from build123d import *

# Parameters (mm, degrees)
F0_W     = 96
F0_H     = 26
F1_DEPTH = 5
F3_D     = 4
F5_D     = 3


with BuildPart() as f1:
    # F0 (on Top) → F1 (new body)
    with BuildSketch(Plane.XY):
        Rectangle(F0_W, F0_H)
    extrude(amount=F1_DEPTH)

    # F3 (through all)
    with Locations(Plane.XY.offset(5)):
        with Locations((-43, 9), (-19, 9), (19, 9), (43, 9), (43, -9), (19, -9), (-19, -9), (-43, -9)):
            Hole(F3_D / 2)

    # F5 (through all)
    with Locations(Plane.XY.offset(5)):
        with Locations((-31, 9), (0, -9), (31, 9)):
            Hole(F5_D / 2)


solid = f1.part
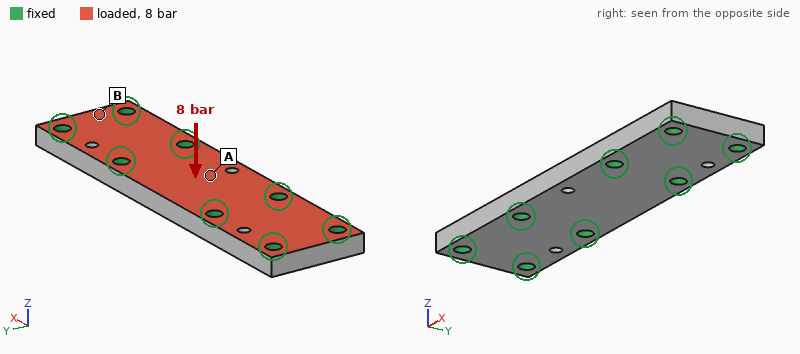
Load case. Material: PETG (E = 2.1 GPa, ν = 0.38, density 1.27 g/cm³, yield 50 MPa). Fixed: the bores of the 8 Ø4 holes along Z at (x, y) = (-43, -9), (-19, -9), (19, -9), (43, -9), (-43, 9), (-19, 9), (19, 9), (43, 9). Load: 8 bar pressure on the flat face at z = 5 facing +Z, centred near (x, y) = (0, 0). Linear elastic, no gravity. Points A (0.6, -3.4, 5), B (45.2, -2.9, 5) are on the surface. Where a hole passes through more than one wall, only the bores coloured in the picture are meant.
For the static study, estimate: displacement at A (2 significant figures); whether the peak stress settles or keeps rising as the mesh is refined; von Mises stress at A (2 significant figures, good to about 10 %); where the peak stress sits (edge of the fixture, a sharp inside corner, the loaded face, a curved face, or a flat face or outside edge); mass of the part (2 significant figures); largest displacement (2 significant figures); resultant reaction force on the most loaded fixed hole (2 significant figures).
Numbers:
0.21 mm
keeps rising
9.7 MPa
edge of the fixture
15 g
0.23 mm
320 N
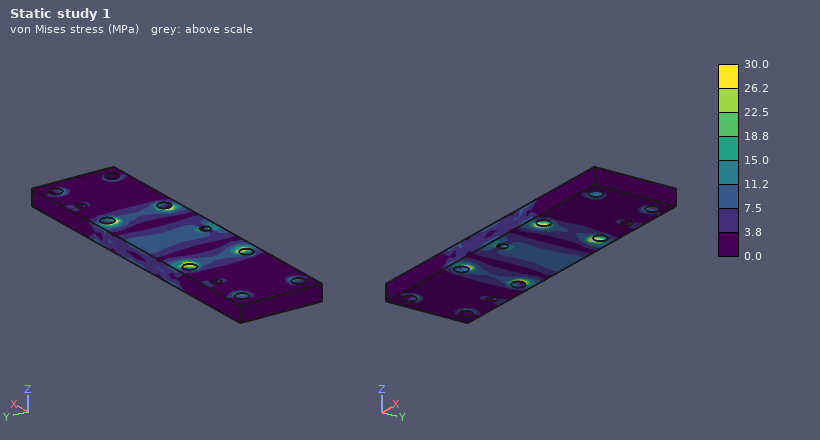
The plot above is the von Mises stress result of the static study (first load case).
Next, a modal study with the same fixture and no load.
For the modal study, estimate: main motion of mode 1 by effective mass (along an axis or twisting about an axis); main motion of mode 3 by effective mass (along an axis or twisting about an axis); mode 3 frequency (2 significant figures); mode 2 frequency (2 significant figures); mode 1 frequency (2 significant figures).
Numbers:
along Z
along Y
9100 Hz
5900 Hz
4300 Hz
